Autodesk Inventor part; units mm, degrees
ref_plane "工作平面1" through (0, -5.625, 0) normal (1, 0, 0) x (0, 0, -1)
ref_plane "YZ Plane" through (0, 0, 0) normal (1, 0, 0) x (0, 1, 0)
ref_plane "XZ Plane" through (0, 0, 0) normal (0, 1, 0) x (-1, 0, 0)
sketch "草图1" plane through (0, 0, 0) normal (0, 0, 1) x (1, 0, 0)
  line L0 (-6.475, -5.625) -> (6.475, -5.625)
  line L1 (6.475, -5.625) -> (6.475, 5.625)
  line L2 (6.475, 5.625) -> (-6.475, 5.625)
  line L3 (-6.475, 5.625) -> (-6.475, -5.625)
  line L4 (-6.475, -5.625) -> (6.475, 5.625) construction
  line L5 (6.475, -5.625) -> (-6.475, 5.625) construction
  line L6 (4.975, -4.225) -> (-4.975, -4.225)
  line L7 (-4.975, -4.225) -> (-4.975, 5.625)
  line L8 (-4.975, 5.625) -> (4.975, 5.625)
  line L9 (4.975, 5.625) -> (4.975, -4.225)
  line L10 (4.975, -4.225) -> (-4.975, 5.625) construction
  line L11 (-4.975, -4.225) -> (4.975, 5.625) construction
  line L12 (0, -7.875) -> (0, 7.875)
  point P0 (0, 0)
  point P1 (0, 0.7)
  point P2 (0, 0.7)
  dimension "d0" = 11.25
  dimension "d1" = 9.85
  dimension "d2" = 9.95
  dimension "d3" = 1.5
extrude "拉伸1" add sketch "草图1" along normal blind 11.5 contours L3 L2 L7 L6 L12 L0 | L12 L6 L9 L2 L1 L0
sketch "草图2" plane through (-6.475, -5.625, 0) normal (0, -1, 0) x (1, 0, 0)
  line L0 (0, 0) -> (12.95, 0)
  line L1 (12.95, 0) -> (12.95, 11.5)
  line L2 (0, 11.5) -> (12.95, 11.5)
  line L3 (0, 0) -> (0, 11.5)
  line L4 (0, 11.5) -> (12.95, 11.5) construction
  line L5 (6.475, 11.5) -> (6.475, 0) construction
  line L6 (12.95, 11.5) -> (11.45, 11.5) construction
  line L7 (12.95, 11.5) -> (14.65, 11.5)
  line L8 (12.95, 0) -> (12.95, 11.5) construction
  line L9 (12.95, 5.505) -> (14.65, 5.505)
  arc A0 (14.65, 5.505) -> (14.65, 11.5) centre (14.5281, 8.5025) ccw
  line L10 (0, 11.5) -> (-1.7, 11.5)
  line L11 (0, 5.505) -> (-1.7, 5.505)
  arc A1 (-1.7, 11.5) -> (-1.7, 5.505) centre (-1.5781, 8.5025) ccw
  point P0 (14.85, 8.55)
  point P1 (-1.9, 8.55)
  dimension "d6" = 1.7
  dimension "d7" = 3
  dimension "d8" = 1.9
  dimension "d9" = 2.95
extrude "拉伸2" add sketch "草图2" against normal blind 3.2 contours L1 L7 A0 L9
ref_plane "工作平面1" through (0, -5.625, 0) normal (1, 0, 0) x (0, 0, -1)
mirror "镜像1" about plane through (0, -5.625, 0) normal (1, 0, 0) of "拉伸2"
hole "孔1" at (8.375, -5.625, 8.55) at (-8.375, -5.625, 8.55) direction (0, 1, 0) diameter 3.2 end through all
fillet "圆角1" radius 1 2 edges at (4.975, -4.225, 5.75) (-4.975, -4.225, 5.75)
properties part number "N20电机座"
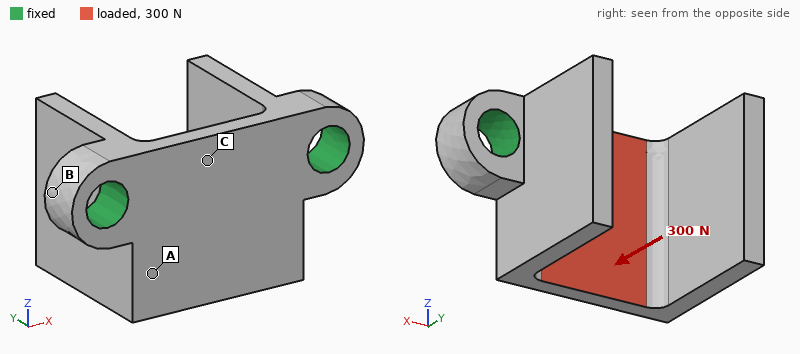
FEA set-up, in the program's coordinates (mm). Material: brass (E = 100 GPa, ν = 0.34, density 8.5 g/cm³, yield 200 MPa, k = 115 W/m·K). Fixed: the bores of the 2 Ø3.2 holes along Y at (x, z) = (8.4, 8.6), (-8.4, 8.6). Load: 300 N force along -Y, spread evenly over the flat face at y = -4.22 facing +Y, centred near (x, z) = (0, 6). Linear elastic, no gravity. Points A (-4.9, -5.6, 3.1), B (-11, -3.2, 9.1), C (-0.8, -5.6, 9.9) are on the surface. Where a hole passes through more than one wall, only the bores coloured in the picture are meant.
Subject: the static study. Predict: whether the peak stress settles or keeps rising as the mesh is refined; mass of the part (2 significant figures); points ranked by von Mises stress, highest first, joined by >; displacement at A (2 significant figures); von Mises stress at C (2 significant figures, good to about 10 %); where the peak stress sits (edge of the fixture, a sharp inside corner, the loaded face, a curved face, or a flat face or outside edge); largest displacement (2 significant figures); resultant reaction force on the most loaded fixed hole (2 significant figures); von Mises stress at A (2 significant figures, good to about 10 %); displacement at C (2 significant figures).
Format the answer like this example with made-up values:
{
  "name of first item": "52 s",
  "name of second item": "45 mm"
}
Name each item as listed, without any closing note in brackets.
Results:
{
  "whether the peak stress settles or keeps rising as the mesh is refined": "keeps rising",
  "mass of the part": "5.5 g",
  "points ranked by von Mises stress, highest first, joined by >": "C > A > B",
  "displacement at A": "5.3 µm",
  "von Mises stress at C": "50 MPa",
  "where the peak stress sits": "edge of the fixture",
  "largest displacement": "16 µm",
  "resultant reaction force on the most loaded fixed hole": "170 N",
  "von Mises stress at A": "24 MPa",
  "displacement at C": "5.8 µm"
}
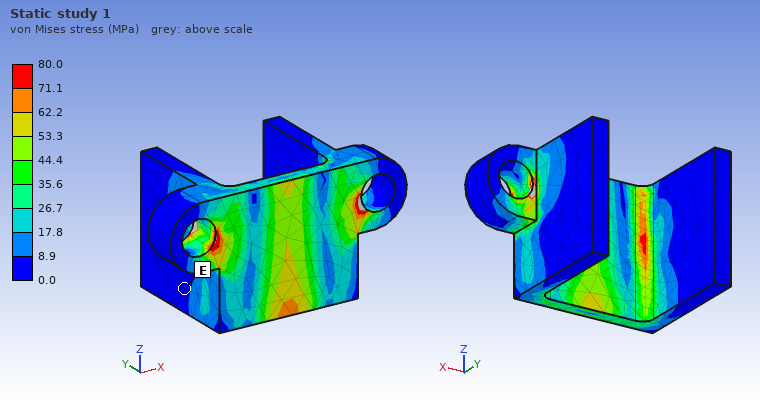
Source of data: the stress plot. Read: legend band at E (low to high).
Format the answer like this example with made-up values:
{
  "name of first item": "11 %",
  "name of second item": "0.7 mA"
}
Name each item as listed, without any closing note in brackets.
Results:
{
  "legend band at E": "0.0 to 8.9 MPa"
}
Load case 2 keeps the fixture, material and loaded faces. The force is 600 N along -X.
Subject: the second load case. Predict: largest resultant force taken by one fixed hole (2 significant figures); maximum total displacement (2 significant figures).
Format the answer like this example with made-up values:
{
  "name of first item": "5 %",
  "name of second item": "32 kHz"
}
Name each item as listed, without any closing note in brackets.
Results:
{
  "largest resultant force taken by one fixed hole": "320 N",
  "maximum total displacement": "3.9 µm"
}
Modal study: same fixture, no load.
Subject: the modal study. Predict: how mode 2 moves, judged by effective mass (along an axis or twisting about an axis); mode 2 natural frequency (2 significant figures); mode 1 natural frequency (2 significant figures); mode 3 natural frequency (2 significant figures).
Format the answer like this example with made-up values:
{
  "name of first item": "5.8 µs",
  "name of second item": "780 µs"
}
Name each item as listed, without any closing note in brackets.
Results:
{
  "how mode 2 moves, judged by effective mass": "along X",
  "mode 2 natural frequency": "9400 Hz",
  "mode 1 natural frequency": "8900 Hz",
  "mode 3 natural frequency": "15 kHz"
}
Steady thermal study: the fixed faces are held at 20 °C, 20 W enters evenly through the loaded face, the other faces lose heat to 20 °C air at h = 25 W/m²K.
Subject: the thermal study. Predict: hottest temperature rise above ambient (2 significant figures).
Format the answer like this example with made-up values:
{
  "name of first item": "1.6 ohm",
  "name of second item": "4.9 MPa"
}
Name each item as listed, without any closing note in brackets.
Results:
{
  "hottest temperature rise above ambient": "35 K"
}
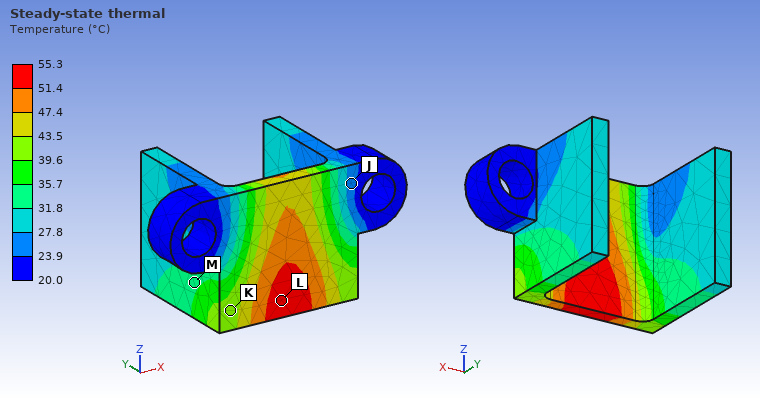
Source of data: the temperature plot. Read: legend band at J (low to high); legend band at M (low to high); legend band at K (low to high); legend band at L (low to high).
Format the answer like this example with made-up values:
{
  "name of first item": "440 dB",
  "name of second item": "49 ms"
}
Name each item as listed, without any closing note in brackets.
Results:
{
  "legend band at J": "23.9 to 27.8 °C",
  "legend band at M": "31.8 to 35.7 °C",
  "legend band at K": "39.6 to 43.5 °C",
  "legend band at L": "51.4 to 55.3 °C"
}
